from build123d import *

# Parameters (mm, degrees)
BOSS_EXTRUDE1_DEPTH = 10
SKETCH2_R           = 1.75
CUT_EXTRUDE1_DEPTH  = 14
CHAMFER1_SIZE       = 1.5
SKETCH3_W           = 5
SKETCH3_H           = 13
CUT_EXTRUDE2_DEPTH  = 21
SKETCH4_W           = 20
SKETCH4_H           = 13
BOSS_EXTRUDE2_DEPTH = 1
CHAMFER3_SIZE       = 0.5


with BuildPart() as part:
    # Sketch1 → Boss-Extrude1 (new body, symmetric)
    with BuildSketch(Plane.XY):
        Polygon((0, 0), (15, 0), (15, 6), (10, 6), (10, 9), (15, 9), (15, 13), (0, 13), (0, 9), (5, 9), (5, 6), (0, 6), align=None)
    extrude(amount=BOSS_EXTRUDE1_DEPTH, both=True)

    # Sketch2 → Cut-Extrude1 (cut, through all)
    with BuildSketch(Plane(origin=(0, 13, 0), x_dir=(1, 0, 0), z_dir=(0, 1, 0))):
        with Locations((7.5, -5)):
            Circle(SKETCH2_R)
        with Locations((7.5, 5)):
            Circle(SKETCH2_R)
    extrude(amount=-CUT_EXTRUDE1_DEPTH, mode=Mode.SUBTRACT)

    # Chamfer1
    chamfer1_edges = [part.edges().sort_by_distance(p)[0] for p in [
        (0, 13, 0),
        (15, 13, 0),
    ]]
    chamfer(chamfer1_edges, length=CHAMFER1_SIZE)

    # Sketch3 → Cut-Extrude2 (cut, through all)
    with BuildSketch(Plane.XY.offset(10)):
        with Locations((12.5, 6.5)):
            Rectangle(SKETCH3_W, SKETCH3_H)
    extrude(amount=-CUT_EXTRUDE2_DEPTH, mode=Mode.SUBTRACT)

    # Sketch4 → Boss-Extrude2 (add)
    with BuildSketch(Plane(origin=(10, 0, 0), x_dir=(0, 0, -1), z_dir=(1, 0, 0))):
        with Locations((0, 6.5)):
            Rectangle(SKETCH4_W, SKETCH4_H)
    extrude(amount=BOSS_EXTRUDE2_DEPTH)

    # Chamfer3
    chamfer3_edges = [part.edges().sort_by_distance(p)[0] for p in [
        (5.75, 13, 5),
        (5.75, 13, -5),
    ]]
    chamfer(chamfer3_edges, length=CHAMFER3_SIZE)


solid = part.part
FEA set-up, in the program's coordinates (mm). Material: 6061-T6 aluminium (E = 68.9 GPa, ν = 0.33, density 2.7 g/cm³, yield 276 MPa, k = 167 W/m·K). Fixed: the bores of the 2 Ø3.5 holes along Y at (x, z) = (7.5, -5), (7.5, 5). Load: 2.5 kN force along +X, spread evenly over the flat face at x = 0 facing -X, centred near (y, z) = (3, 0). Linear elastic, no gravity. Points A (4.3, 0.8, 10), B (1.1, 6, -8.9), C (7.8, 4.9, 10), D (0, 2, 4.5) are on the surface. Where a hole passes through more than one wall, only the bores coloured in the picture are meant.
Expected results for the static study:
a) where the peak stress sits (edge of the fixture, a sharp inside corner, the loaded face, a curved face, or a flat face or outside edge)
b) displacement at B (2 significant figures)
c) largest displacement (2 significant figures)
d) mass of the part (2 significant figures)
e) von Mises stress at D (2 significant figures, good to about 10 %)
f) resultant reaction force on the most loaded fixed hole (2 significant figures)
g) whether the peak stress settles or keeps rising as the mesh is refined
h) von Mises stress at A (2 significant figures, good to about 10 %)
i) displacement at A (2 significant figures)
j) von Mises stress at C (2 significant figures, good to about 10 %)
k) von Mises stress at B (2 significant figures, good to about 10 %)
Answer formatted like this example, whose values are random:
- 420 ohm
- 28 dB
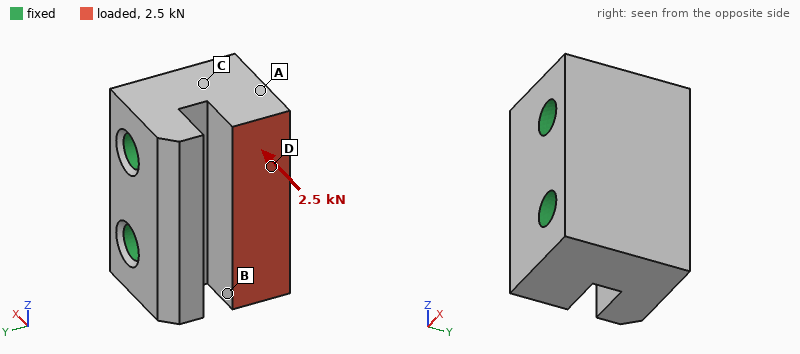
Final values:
- edge of the fixture
- 2.4 µm
- 3.4 µm
- 6.2 g
- 25 MPa
- 1.3 kN
- keeps rising
- 13 MPa
- 2.0 µm
- 9.5 MPa
- 21 MPa
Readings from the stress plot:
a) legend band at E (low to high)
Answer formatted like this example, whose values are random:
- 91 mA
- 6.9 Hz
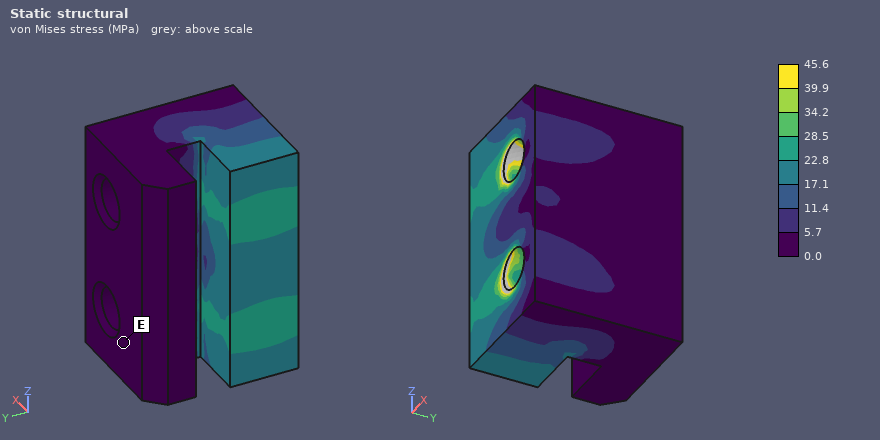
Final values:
- 0.0 to 5.7 MPa
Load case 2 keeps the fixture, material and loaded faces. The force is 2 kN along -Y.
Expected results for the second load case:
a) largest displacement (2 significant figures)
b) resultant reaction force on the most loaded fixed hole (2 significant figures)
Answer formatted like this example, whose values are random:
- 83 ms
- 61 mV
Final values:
- 14 µm
- 1.0 kN
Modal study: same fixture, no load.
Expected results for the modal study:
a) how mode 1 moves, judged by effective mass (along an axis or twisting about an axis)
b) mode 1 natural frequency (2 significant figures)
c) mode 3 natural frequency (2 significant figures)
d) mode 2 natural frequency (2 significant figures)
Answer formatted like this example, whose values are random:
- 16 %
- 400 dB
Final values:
- along Y
- 68 kHz
- 79 kHz
- 76 kHz
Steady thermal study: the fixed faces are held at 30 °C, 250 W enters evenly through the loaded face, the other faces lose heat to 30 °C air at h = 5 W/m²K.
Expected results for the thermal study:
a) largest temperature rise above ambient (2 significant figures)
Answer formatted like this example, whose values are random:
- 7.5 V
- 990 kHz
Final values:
- 84 K
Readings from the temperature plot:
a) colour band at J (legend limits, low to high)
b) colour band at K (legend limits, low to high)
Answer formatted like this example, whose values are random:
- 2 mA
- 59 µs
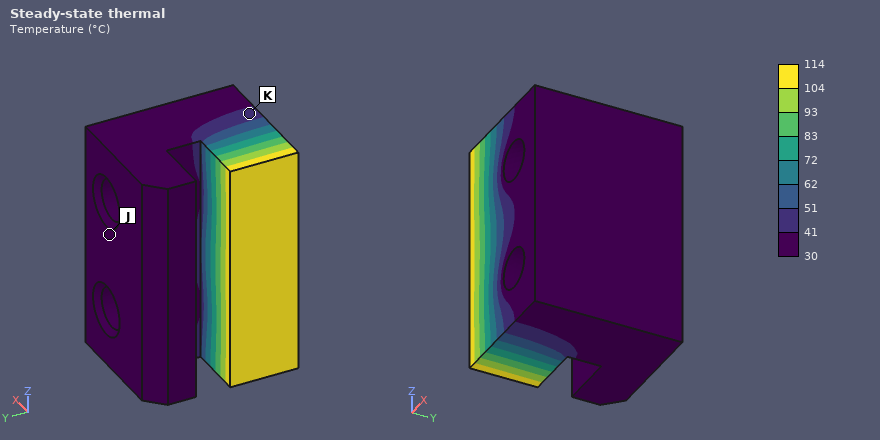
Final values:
- 30 to 41 °C
- 41 to 51 °C
